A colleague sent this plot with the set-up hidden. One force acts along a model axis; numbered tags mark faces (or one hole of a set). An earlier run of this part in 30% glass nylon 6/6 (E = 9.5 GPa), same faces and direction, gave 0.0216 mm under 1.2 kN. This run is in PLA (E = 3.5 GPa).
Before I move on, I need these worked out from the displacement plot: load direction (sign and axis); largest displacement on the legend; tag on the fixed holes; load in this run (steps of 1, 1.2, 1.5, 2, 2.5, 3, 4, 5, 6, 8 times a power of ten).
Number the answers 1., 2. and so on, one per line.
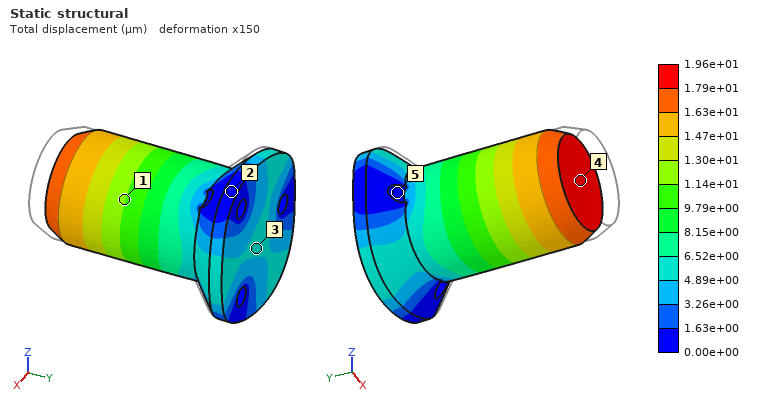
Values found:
1. +Y
2. 1.96e+01 µm
3. 5
4. 400 N
